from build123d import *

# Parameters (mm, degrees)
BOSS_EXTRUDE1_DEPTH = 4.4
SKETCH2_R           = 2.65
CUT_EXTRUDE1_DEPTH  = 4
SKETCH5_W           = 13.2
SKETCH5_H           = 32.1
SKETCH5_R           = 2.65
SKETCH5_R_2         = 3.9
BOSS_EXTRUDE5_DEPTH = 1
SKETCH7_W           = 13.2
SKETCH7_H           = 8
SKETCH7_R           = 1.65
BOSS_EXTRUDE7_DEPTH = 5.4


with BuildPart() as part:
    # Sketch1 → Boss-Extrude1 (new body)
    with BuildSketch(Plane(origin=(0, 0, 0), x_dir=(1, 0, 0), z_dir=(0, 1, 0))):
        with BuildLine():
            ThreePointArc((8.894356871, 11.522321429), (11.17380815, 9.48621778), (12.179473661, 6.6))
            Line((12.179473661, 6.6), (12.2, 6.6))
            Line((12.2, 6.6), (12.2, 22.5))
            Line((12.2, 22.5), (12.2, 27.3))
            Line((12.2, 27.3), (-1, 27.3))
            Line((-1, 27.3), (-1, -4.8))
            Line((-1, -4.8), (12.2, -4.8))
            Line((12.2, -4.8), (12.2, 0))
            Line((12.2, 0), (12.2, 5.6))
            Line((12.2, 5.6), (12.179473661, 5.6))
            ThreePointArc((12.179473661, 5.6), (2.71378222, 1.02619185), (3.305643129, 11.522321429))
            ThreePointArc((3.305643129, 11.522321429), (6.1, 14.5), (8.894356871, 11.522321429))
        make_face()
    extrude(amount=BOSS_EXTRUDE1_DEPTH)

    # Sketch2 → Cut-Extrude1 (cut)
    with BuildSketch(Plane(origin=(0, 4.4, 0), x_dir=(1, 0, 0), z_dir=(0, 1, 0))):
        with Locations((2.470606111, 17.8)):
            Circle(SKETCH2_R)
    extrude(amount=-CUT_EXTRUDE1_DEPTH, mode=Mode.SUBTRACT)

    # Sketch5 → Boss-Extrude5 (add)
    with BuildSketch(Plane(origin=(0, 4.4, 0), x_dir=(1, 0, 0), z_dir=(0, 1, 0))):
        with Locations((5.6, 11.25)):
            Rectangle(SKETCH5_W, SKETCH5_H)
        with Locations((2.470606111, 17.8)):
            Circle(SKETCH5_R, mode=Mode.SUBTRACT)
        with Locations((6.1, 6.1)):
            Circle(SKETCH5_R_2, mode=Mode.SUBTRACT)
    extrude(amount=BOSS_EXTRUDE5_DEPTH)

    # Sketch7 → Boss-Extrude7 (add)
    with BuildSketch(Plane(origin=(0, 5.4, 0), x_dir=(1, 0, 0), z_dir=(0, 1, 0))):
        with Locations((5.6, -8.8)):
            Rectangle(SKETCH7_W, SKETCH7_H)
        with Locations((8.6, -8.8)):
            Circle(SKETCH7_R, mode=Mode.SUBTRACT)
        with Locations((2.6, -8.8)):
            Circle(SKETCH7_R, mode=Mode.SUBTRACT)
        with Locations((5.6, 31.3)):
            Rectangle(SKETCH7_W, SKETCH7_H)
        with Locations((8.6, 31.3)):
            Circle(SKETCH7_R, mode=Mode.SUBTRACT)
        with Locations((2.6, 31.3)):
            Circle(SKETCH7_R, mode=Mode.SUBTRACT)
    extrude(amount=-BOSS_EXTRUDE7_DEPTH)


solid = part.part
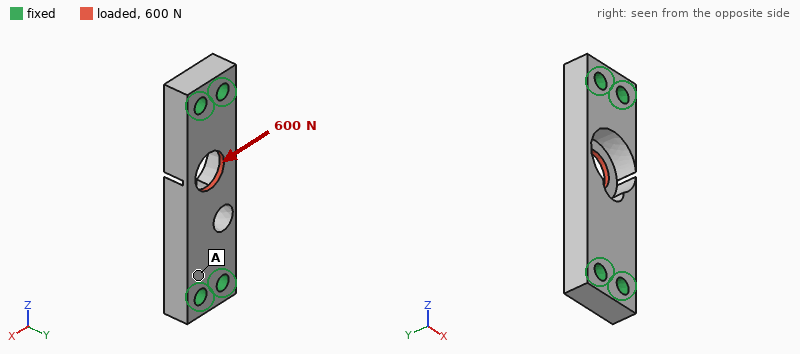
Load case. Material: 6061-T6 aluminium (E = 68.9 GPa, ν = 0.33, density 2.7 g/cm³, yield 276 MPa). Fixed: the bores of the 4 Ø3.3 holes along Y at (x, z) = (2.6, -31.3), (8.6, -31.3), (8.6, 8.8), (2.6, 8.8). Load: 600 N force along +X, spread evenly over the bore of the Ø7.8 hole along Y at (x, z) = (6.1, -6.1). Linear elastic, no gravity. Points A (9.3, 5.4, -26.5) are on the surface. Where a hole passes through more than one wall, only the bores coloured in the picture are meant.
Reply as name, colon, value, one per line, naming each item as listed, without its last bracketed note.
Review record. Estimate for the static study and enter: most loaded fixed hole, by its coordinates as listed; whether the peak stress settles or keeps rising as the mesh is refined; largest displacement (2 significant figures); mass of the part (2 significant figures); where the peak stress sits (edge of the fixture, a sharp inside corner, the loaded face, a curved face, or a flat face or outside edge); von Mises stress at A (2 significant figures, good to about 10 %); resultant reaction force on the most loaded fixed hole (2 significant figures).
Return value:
most loaded fixed hole, by its coordinates as listed: (8.6, -31.3)
whether the peak stress settles or keeps rising as the mesh is refined: keeps rising
largest displacement: 20 µm
mass of the part: 6.8 g
where the peak stress sits: a sharp inside corner
von Mises stress at A: 11 MPa
resultant reaction force on the most loaded fixed hole: 470 N
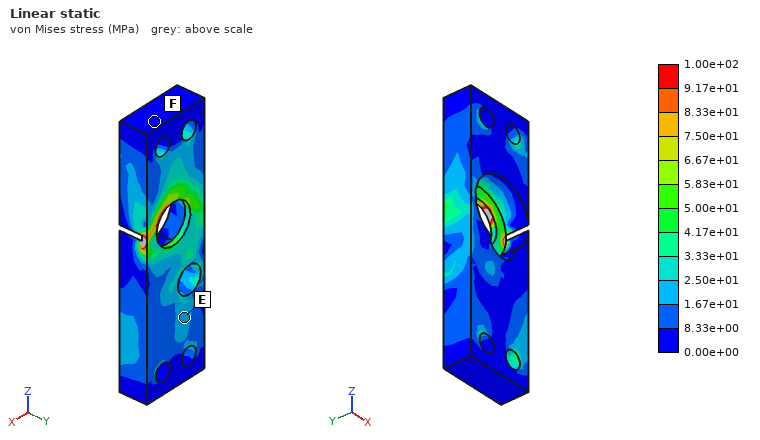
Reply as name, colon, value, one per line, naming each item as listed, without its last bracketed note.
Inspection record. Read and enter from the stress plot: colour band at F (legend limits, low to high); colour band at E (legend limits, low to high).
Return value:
colour band at F: 0.00e+00 to 8.33e+00 MPa
colour band at E: 1.67e+01 to 2.50e+01 MPa
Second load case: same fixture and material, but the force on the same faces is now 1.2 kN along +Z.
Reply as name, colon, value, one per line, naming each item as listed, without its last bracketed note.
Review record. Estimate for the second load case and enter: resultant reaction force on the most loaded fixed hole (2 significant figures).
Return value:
resultant reaction force on the most loaded fixed hole: 360 N
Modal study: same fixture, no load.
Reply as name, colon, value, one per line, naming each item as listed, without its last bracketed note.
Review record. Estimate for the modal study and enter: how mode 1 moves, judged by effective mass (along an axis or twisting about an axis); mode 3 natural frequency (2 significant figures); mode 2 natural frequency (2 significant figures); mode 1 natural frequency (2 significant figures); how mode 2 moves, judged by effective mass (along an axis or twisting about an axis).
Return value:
how mode 1 moves, judged by effective mass: along Y
mode 3 natural frequency: 28 kHz
mode 2 natural frequency: 26 kHz
mode 1 natural frequency: 17 kHz
how mode 2 moves, judged by effective mass: along X
